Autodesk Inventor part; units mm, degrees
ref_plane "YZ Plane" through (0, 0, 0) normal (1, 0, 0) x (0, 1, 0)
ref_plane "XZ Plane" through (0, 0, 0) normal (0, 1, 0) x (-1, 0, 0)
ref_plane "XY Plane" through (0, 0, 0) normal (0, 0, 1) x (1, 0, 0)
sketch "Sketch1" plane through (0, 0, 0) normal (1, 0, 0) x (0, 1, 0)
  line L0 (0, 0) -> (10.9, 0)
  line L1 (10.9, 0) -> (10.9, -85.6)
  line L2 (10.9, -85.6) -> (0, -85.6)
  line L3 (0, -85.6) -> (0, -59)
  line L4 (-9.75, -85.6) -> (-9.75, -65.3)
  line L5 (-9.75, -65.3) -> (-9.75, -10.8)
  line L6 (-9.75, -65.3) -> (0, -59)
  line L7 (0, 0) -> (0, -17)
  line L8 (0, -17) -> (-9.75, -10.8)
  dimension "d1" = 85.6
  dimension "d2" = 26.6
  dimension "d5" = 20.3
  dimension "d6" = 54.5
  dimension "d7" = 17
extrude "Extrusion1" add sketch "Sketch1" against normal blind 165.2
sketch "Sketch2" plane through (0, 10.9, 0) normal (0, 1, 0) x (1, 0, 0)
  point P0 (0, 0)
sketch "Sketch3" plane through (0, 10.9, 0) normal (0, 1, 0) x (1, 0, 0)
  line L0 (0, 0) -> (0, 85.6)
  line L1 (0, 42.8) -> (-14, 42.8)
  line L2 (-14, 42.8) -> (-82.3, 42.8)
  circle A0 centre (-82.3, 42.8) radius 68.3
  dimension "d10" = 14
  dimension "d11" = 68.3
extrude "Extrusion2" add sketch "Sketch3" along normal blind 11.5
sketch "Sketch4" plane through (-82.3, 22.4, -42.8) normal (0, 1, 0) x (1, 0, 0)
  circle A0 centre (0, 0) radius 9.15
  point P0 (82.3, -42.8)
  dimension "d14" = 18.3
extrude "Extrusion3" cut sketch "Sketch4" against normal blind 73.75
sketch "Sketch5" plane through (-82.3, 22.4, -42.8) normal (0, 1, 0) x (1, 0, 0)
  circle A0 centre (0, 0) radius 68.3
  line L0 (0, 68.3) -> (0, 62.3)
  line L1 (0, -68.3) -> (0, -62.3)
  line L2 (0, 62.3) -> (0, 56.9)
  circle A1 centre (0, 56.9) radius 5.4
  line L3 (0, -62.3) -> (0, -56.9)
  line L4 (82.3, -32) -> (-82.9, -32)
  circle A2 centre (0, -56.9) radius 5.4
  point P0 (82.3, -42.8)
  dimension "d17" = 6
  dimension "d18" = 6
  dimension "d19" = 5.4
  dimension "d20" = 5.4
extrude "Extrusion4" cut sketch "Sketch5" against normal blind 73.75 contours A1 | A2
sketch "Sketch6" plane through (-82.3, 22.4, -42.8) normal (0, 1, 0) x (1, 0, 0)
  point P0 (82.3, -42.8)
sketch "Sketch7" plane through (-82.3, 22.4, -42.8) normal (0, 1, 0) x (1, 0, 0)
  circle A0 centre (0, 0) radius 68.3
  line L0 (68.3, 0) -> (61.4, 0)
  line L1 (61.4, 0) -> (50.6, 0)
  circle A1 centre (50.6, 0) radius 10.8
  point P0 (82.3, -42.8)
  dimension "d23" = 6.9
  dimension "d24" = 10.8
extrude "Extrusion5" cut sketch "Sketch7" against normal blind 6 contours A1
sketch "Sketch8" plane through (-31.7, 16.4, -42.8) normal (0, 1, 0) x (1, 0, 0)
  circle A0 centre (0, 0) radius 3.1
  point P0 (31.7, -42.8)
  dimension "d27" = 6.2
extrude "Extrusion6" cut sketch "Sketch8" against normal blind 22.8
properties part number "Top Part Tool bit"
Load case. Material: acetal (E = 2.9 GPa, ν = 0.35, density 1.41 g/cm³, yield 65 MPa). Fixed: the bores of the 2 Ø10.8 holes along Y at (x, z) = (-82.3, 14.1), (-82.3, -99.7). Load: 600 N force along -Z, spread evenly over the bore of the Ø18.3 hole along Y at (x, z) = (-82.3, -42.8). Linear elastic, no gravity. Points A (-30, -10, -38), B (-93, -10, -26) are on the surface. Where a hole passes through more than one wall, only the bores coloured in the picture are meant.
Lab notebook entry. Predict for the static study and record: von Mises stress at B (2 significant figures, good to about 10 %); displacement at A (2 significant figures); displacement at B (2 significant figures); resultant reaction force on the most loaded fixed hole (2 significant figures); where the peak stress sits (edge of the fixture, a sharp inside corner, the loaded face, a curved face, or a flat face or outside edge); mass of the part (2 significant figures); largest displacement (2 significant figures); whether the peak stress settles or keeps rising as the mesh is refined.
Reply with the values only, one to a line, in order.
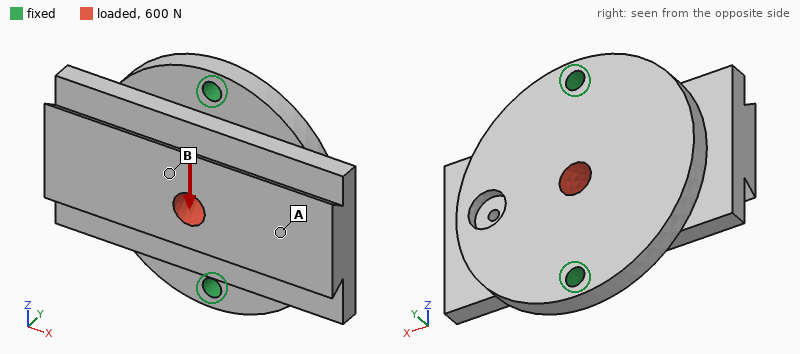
0.22 MPa
7.5 µm
10 µm
310 N
edge of the fixture
550 g
13 µm
keeps rising
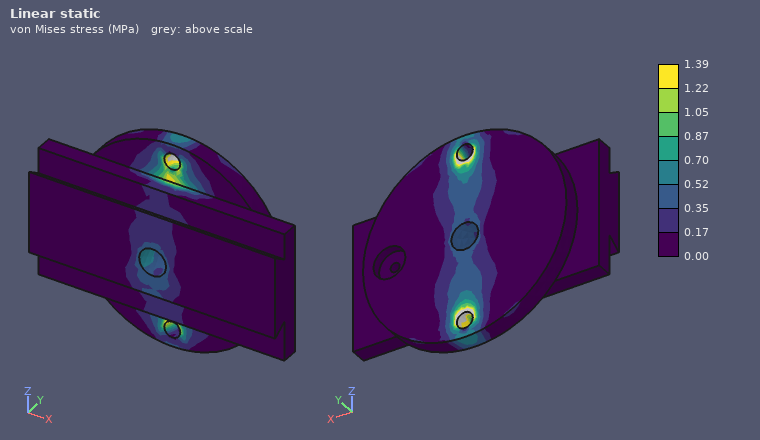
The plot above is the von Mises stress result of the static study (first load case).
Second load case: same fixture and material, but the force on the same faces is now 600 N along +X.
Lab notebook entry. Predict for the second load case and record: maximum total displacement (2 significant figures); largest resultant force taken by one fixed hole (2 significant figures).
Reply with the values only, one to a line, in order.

0.16 mm
300 N
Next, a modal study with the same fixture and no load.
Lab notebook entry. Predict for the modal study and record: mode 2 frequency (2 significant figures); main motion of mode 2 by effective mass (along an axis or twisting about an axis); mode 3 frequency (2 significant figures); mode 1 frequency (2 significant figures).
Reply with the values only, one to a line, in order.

740 Hz
along Y
1600 Hz
290 Hz
